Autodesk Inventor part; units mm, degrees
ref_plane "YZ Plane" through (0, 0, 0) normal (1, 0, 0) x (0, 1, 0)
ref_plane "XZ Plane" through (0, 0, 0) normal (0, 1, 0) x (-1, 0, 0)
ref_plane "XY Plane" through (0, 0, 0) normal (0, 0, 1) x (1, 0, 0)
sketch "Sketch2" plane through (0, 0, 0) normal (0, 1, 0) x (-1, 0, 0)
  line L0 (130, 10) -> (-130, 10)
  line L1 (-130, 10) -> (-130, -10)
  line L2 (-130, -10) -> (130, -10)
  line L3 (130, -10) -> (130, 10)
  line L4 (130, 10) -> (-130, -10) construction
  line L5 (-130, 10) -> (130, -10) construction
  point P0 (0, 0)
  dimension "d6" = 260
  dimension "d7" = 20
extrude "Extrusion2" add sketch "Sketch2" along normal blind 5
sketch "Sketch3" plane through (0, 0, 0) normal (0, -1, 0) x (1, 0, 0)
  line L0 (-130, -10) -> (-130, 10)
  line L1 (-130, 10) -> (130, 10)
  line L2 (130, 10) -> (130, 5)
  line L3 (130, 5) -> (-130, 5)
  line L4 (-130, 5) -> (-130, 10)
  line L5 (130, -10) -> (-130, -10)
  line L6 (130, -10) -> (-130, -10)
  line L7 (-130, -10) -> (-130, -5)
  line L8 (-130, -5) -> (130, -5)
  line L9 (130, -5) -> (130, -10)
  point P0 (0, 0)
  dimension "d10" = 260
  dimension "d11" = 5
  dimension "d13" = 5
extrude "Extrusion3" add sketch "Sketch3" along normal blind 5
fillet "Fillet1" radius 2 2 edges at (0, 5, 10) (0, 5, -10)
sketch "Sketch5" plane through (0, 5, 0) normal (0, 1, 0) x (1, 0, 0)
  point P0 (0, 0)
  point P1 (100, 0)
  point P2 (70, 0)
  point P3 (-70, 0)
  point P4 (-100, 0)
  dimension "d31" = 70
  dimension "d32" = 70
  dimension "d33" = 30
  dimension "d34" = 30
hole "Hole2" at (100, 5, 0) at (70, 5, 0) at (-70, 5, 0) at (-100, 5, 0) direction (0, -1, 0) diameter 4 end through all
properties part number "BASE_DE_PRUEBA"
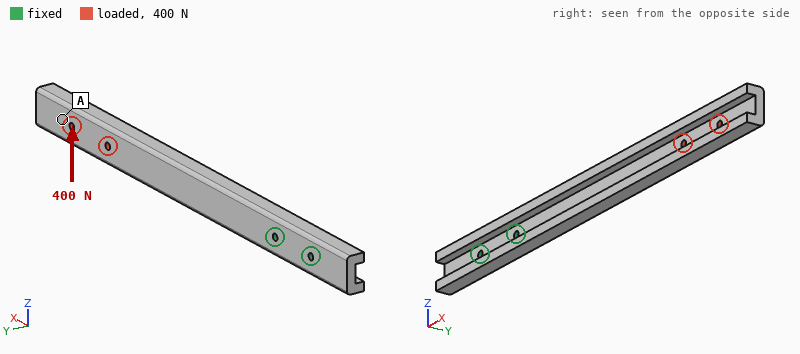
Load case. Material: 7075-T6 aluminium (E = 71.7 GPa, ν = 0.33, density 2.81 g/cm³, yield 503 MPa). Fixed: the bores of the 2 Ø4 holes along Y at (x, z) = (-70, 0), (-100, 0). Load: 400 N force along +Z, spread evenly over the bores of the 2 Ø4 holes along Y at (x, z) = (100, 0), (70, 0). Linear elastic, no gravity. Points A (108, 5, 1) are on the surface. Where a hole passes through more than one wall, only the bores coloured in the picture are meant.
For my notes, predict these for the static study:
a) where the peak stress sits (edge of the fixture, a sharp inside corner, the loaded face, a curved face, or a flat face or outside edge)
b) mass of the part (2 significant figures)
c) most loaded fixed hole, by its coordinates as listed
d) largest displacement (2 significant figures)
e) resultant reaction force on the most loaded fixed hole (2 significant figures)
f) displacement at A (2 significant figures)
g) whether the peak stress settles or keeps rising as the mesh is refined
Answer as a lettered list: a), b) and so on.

a) edge of the fixture
b) 110 g
c) (-70, 0)
d) 2.1 mm
e) 2.0 kN
f) 1.8 mm
g) keeps rising
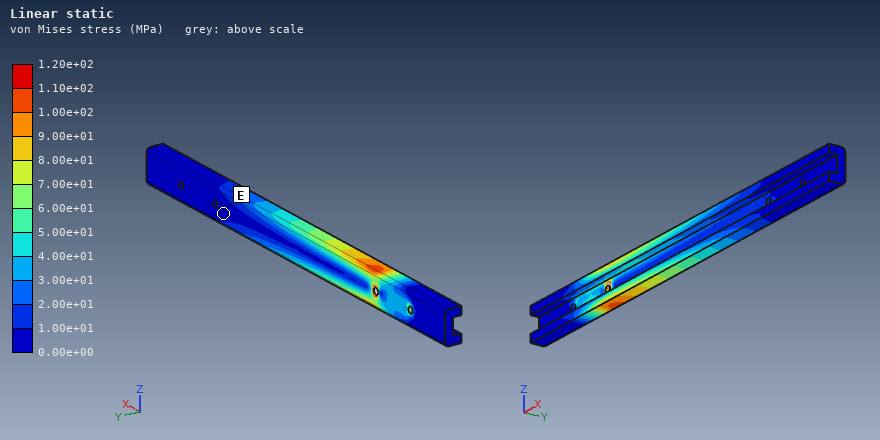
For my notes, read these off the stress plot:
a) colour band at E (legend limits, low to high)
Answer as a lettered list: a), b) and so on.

a) 0.00e+00 to 1.00e+01 MPa
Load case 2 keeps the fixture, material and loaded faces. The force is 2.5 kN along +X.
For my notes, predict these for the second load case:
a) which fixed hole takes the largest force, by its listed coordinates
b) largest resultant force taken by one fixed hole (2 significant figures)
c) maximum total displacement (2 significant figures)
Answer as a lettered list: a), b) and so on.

a) (-70, 0)
b) 2.1 kN
c) 1.00 mm
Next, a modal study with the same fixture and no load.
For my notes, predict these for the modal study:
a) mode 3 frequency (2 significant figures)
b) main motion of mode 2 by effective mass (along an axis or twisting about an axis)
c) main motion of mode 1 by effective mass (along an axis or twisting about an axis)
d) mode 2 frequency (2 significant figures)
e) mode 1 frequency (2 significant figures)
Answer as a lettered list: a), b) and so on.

a) 1100 Hz
b) along Z
c) along Y
d) 400 Hz
e) 190 Hz
